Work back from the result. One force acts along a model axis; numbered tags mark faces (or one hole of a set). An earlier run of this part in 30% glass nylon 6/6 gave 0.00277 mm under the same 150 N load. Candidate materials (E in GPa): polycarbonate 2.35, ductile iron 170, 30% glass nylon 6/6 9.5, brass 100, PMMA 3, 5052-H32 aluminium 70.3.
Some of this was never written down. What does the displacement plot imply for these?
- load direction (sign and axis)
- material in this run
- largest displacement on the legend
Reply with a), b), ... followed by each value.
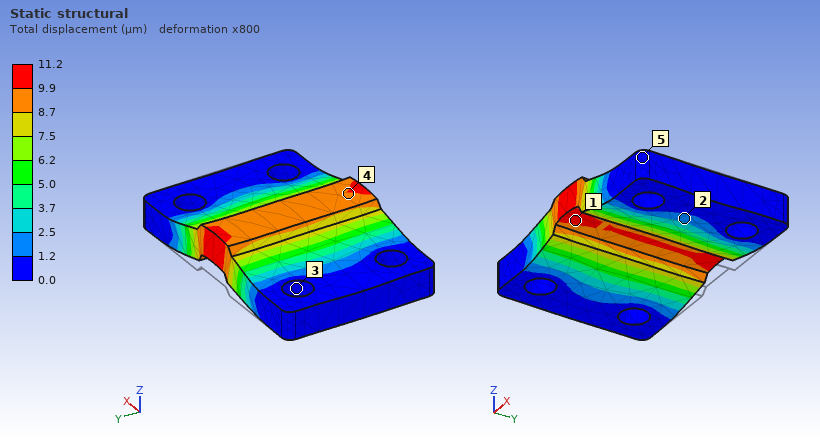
a) +Z
b) polycarbonate
c) 11.2 µm
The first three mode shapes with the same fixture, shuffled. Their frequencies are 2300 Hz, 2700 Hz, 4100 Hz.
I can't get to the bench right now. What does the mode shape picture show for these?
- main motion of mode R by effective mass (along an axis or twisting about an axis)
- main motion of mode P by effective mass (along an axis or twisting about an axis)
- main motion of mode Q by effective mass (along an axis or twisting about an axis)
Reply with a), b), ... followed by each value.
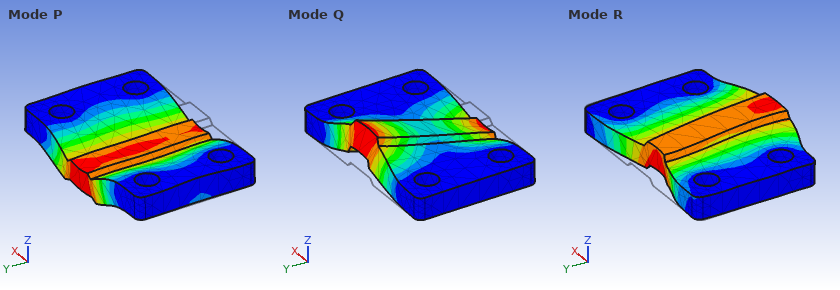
a) along Y
b) along Z
c) twisting about X
